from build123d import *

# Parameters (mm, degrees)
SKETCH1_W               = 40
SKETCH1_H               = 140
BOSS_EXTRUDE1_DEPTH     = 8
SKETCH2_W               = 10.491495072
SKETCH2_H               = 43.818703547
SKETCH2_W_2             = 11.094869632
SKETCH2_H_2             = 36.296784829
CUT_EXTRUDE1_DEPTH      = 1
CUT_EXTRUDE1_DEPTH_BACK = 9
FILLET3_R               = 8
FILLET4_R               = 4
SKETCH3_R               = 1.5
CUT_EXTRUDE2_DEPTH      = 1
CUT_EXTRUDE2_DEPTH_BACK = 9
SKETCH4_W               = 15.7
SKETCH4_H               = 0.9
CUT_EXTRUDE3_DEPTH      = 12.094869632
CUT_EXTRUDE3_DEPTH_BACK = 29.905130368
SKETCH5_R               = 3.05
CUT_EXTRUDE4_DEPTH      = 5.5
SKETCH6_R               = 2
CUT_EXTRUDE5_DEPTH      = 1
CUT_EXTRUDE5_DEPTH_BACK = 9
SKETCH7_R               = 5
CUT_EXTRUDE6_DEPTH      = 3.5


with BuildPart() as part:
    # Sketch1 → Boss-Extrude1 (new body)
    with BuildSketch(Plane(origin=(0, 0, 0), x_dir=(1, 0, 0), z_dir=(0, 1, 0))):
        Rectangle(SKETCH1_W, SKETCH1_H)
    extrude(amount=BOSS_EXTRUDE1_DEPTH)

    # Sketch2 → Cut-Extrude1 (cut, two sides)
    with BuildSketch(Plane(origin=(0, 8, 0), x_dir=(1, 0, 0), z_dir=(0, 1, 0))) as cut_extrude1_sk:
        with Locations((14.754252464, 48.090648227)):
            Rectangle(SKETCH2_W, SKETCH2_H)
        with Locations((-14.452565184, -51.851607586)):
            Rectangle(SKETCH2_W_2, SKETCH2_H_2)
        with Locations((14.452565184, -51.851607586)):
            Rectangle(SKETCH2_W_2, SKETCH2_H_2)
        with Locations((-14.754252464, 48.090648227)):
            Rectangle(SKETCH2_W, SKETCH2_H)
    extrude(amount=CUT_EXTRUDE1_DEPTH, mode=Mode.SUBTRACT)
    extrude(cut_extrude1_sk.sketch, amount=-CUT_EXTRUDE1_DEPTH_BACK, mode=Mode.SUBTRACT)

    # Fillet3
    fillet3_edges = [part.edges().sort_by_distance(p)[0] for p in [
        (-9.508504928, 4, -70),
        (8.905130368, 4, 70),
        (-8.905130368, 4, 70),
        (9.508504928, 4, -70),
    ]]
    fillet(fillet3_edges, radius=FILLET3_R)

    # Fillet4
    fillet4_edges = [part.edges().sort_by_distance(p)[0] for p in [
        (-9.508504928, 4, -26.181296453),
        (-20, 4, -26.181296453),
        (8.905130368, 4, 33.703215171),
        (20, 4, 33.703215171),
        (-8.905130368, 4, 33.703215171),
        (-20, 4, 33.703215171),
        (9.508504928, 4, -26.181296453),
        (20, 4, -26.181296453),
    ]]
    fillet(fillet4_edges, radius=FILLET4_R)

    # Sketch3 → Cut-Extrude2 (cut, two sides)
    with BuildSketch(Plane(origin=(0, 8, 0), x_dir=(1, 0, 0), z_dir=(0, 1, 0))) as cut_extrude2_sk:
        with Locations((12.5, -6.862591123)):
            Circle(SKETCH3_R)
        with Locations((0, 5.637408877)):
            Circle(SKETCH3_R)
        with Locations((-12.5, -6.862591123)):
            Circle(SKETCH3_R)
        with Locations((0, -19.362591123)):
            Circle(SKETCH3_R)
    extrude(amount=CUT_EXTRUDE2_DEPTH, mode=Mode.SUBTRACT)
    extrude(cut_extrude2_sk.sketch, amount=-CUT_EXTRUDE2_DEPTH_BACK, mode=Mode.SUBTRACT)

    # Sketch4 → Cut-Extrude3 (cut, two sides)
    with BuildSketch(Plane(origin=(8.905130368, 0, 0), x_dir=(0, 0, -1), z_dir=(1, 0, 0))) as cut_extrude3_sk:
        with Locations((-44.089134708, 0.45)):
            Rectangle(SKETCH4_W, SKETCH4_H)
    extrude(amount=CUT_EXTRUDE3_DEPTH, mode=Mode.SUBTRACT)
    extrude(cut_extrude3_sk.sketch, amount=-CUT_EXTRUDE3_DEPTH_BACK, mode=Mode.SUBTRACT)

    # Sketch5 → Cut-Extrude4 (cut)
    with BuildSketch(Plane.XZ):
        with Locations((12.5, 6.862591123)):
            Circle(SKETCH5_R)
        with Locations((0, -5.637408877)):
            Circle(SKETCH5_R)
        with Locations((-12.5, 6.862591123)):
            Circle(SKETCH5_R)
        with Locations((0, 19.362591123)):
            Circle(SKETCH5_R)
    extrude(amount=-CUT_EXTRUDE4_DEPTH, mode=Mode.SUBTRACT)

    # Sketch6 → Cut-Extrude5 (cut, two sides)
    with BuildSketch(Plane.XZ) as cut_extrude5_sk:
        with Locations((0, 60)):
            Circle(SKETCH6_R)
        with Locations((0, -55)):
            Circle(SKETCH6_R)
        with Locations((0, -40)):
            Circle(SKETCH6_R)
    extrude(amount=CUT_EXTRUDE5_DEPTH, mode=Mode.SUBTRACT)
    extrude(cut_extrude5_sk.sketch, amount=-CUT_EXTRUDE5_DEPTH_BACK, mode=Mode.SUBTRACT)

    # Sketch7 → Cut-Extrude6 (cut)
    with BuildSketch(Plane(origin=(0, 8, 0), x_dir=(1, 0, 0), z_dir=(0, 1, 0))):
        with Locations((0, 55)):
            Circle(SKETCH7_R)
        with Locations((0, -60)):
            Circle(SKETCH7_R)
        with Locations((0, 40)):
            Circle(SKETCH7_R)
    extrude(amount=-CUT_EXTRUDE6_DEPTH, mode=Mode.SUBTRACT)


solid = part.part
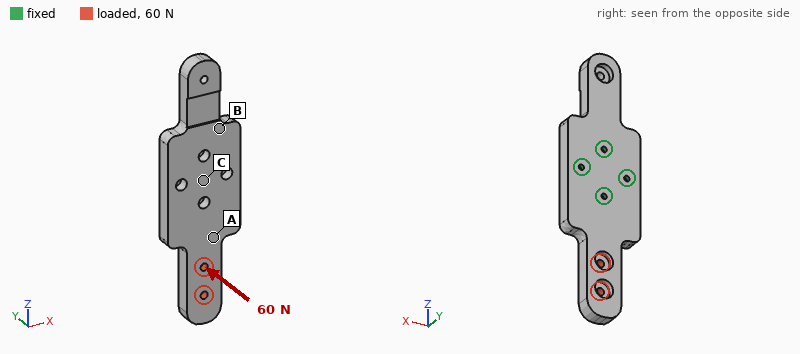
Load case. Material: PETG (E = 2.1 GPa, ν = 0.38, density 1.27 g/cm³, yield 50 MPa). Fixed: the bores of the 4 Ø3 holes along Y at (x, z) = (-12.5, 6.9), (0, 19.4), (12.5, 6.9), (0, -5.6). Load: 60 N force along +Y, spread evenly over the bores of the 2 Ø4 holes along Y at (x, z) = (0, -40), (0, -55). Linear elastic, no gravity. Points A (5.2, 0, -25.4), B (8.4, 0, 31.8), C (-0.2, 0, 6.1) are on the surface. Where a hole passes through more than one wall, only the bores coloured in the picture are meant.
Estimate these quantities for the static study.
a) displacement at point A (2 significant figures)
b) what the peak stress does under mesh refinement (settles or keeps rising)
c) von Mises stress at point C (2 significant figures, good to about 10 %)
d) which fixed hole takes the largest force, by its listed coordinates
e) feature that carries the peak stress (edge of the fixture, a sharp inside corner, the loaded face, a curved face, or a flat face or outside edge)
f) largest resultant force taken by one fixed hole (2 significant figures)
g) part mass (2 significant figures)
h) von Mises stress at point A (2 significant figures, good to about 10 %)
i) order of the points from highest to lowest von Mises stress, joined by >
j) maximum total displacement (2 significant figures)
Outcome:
0.28 mm
keeps rising
1.6 MPa
(0, -5.6)
edge of the fixture
220 N
36 g
5.3 MPa
A > C > B
1.5 mm
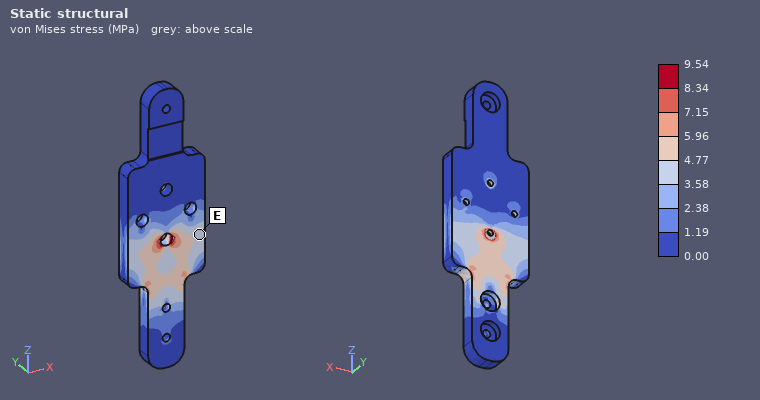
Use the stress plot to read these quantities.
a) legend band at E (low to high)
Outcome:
3.58 to 4.77 MPa
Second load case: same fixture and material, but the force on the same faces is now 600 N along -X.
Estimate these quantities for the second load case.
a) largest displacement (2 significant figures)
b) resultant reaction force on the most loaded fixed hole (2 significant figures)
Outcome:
1.7 mm
780 N
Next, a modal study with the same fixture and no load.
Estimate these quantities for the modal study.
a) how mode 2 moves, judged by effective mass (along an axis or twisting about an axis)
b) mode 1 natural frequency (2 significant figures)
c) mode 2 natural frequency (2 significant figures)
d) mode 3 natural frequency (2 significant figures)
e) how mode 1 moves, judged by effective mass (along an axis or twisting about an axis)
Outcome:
along Y
450 Hz
690 Hz
1300 Hz
along Y
